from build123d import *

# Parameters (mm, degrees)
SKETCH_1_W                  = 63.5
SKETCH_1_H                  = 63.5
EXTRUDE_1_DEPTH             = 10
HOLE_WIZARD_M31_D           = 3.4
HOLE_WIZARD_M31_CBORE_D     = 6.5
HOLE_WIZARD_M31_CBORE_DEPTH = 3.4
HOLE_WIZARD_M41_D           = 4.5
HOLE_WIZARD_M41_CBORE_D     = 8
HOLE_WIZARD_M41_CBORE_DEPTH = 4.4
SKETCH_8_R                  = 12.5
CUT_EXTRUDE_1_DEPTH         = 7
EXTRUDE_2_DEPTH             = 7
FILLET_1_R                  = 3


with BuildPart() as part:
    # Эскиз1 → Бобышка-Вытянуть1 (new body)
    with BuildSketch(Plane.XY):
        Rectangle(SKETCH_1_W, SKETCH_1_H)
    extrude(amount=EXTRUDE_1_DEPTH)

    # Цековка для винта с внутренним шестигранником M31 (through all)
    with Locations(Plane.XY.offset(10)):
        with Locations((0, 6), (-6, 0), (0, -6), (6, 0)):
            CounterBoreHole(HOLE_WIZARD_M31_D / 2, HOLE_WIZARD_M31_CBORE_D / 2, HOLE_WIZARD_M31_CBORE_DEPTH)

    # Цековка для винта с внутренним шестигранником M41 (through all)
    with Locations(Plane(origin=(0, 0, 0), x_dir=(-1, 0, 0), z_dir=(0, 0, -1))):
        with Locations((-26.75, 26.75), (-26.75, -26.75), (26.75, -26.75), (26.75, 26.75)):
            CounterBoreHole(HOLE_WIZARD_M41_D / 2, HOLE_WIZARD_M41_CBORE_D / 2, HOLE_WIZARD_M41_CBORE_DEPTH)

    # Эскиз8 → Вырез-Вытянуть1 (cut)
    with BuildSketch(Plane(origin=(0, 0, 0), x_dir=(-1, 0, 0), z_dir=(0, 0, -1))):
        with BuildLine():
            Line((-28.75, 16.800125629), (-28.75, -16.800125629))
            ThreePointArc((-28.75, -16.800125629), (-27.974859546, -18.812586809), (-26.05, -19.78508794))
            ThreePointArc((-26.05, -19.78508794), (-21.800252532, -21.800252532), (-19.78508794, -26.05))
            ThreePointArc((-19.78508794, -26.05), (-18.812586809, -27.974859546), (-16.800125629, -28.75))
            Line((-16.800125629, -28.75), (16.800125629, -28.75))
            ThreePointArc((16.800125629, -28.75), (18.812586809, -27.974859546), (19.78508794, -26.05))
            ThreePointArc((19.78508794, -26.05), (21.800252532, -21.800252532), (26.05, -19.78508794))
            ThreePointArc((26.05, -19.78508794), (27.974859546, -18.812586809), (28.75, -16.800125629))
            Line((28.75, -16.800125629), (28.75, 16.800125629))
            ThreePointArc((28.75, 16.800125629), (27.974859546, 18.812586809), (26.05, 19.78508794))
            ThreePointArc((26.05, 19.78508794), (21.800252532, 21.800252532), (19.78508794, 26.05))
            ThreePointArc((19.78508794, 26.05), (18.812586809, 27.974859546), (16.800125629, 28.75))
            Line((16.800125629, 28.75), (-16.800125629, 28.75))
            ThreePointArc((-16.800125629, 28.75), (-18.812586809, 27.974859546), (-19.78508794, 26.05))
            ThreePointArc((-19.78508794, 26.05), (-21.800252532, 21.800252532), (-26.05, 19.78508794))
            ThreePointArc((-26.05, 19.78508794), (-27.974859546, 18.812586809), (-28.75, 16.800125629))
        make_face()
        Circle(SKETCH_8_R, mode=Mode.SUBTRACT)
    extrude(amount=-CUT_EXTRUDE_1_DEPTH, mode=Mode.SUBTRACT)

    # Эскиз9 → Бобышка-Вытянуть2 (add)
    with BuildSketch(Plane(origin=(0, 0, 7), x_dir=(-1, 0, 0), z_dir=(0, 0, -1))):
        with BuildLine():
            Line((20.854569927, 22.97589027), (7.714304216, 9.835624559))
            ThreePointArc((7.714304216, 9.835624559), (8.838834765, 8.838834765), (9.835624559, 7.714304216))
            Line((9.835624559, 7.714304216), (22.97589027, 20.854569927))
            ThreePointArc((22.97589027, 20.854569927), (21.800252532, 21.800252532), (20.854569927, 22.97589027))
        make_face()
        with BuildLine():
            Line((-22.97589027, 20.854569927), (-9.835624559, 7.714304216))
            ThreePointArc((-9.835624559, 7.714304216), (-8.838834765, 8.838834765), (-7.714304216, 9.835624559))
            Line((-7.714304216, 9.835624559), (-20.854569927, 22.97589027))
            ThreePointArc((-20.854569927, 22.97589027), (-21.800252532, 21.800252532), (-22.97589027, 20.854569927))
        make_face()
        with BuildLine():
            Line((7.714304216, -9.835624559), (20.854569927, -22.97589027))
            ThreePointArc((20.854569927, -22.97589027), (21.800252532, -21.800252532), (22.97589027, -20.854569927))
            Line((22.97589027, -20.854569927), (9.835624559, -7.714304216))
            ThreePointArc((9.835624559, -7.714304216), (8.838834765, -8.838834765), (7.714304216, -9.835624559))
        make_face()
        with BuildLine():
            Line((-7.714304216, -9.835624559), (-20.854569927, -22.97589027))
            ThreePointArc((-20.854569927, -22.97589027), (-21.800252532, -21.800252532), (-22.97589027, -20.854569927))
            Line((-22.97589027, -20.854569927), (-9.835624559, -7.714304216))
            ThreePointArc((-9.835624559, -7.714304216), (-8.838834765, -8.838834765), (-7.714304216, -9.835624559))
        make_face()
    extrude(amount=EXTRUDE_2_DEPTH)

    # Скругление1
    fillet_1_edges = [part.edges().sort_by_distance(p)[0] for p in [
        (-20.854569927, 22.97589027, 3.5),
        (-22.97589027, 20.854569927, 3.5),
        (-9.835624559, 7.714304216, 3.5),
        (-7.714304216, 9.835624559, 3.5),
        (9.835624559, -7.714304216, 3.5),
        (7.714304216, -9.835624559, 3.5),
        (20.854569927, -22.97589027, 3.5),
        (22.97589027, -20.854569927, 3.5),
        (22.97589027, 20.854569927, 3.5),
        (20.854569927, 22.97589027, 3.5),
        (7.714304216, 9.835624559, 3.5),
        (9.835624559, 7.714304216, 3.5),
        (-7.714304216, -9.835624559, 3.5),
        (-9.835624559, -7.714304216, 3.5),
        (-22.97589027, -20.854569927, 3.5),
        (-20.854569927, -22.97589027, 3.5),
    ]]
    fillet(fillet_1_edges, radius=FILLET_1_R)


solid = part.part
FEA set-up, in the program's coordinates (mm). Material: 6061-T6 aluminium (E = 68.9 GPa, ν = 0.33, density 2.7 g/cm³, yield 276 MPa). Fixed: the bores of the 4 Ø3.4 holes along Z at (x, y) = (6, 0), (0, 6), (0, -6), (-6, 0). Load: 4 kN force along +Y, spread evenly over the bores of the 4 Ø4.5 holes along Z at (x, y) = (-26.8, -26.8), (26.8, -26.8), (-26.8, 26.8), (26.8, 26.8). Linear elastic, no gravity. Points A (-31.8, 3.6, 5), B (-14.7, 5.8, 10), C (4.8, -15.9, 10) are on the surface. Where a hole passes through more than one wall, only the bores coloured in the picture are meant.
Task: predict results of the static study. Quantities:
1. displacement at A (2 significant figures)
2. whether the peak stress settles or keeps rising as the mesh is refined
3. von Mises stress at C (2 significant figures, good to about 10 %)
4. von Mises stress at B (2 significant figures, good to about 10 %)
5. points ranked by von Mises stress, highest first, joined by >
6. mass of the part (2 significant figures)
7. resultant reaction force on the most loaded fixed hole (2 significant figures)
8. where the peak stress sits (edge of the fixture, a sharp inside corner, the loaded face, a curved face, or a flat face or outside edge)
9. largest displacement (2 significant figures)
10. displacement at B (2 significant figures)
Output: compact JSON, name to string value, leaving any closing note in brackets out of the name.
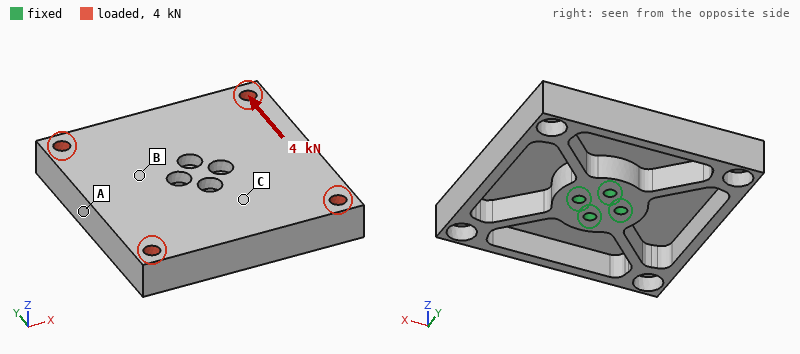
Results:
{"displacement at A": "12 µm", "whether the peak stress settles or keeps rising as the mesh is refined": "keeps rising", "von Mises stress at C": "10 MPa", "von Mises stress at B": "19 MPa", "points ranked by von Mises stress, highest first, joined by >": "B > C > A", "mass of the part": "60 g", "resultant reaction force on the most loaded fixed hole": "1.4 kN", "where the peak stress sits": "edge of the fixture", "largest displacement": "21 µm", "displacement at B": "7.0 µm"}
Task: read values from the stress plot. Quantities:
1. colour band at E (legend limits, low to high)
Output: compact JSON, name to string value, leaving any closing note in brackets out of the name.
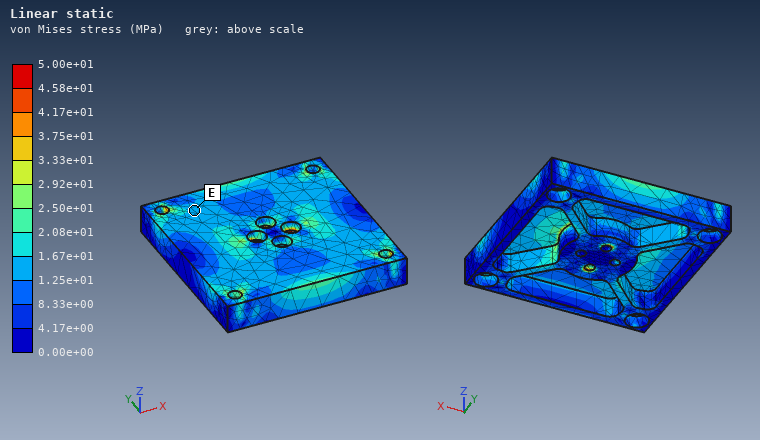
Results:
{"colour band at E": "1.25e+01 to 1.67e+01 MPa"}
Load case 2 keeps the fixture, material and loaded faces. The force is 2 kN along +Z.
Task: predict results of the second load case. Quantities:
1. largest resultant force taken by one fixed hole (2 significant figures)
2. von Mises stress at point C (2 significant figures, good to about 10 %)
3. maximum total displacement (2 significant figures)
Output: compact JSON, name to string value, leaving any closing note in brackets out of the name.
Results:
{"largest resultant force taken by one fixed hole": "640 N", "von Mises stress at point C": "40 MPa", "maximum total displacement": "0.10 mm"}
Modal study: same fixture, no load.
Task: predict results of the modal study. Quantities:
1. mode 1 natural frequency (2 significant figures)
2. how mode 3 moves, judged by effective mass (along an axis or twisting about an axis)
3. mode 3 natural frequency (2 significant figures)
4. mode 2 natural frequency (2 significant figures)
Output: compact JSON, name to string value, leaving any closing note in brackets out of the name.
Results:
{"mode 1 natural frequency": "4100 Hz", "how mode 3 moves, judged by effective mass": "along Z", "mode 3 natural frequency": "4900 Hz", "mode 2 natural frequency": "4100 Hz"}
